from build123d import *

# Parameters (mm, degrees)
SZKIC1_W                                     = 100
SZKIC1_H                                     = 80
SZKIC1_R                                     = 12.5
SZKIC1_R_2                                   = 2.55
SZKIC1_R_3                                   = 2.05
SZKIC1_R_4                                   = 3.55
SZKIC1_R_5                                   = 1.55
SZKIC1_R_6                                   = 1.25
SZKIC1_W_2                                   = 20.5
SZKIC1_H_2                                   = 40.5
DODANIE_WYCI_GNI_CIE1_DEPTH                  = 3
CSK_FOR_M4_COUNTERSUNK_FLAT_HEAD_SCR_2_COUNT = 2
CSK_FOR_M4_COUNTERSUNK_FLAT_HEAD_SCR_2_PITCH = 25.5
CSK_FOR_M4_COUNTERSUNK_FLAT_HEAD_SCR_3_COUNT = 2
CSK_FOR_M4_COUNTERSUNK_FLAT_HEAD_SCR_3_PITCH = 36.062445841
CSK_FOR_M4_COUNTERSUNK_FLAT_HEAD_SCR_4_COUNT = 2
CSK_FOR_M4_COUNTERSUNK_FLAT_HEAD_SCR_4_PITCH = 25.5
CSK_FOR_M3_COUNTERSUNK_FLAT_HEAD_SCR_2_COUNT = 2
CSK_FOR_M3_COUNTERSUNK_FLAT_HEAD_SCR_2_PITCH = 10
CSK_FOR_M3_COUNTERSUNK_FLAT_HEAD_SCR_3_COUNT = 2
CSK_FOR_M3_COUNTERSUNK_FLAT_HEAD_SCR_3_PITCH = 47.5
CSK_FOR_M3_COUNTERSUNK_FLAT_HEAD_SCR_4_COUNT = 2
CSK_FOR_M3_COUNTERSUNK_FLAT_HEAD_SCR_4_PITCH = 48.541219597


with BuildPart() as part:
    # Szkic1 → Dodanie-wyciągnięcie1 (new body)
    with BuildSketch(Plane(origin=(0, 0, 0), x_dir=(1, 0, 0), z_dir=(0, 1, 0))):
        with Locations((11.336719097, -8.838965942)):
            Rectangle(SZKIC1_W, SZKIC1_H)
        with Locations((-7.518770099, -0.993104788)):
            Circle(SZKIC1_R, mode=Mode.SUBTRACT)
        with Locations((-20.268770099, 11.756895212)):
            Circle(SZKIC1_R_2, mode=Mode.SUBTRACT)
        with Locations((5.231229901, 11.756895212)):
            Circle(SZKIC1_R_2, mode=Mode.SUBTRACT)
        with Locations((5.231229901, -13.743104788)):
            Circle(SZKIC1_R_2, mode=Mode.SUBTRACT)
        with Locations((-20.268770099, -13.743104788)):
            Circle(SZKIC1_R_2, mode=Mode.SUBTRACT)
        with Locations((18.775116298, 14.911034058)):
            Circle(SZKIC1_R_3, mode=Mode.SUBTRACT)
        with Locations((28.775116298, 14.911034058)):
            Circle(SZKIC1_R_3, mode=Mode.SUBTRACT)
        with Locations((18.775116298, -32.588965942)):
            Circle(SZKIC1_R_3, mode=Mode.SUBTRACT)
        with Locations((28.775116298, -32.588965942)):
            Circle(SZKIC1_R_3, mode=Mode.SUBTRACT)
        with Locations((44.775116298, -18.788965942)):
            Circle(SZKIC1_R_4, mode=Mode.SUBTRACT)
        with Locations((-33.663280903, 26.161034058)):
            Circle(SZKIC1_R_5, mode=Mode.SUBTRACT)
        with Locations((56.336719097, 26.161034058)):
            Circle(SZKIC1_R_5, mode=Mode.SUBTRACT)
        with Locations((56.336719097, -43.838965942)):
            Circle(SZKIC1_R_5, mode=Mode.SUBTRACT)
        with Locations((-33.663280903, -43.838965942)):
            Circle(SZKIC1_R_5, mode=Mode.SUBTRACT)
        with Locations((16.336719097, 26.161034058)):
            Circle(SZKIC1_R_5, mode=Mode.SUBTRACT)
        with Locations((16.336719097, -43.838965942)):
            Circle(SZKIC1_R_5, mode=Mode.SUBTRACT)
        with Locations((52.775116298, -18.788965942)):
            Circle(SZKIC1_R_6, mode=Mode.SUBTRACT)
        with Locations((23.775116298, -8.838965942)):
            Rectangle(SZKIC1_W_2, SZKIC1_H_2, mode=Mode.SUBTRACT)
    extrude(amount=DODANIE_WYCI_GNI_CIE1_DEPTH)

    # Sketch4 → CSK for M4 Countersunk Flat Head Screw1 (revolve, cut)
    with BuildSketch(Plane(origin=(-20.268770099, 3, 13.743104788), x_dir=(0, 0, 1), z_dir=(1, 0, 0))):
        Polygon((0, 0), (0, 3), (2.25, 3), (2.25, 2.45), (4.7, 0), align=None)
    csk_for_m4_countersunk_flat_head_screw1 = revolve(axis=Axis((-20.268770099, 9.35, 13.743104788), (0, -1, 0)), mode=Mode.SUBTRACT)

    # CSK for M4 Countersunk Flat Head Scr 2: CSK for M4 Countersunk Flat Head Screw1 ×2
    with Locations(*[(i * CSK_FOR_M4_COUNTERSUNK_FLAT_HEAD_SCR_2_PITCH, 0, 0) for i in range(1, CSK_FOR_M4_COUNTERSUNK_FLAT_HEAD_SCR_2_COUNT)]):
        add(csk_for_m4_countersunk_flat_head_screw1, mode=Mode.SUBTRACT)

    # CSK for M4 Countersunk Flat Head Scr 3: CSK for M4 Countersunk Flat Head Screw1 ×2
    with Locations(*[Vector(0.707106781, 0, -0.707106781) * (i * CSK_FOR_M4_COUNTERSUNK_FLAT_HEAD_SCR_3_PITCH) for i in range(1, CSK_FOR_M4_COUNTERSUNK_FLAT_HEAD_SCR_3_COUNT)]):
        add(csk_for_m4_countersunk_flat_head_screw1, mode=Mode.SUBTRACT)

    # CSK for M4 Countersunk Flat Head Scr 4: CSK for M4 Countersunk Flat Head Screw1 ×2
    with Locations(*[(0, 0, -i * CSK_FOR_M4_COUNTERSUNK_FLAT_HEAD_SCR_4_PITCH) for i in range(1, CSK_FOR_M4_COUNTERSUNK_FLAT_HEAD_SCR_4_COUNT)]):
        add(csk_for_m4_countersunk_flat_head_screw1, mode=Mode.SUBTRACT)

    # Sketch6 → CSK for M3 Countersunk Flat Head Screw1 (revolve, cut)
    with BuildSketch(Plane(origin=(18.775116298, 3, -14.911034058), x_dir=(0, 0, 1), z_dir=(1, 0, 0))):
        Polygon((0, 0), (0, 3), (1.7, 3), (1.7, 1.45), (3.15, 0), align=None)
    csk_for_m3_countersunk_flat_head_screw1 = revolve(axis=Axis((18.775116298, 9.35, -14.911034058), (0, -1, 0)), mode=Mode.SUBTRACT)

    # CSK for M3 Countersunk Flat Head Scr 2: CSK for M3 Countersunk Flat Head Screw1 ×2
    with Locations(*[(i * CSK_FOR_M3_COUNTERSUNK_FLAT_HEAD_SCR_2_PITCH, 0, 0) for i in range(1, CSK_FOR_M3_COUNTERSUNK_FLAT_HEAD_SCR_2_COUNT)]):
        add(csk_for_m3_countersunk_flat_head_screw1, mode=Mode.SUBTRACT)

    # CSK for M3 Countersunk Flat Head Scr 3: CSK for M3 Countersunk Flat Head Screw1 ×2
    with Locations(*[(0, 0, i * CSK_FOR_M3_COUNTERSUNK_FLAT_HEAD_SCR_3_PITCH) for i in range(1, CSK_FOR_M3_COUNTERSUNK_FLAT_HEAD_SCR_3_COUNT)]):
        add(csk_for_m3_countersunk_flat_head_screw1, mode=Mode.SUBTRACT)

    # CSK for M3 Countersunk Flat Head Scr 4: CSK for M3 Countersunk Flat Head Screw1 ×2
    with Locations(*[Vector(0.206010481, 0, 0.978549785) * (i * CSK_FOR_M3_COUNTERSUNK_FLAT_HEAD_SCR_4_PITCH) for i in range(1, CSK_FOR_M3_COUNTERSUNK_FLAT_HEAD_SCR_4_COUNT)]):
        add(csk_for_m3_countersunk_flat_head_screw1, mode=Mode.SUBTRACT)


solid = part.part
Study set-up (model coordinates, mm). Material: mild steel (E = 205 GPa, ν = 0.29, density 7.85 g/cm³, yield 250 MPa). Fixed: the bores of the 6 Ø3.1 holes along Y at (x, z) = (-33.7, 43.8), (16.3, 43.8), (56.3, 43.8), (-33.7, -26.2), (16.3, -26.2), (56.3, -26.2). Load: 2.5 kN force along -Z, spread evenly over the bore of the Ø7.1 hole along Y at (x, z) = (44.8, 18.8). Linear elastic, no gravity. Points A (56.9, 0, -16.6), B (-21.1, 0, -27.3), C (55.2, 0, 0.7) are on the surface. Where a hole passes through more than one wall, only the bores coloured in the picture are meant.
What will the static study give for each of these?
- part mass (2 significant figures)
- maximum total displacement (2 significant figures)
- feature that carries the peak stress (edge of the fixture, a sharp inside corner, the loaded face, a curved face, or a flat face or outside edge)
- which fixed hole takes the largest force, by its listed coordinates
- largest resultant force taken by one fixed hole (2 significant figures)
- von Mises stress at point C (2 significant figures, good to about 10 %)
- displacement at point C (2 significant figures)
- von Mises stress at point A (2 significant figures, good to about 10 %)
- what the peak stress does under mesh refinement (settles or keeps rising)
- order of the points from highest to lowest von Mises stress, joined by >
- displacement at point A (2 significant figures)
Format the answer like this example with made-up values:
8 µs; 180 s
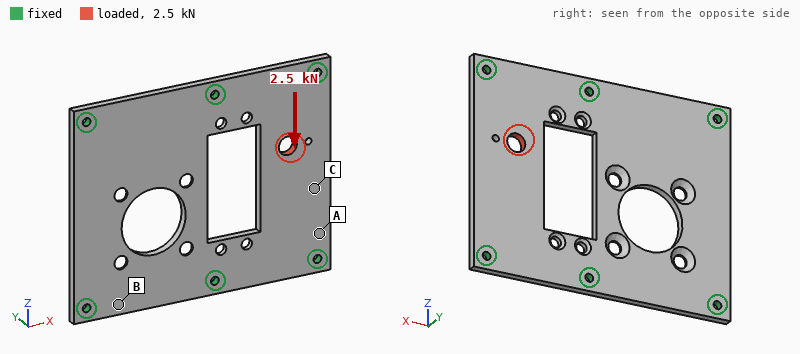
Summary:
150 g; 4.7 µm; edge of the fixture; (56.3, 43.8); 1.2 kN; 12 MPa; 2.3 µm; 19 MPa; keeps rising; A > C > B; 1.1 µm
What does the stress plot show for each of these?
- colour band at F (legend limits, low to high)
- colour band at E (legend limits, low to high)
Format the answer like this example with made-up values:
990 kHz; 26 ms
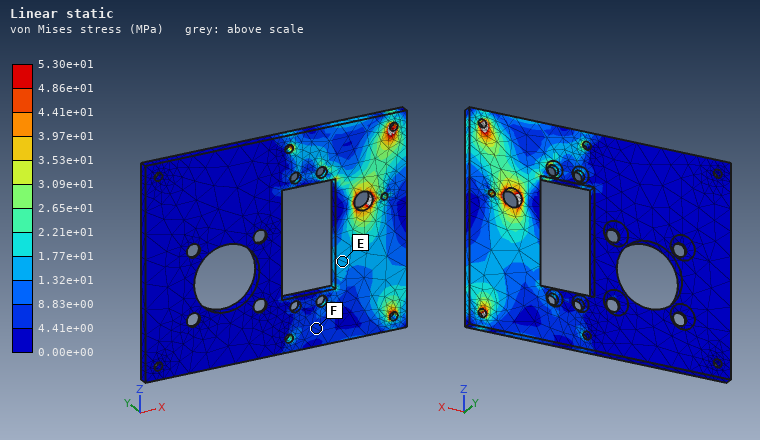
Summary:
4.41e+00 to 8.83e+00 MPa; 1.32e+01 to 1.77e+01 MPa
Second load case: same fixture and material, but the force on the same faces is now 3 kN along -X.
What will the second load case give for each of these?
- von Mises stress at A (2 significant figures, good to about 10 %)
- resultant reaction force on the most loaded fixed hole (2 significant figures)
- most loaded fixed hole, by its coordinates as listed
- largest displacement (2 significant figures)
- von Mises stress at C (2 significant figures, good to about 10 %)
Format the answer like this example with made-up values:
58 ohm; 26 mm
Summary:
19 MPa; 1.3 kN; (56.3, 43.8); 13 µm; 23 MPa
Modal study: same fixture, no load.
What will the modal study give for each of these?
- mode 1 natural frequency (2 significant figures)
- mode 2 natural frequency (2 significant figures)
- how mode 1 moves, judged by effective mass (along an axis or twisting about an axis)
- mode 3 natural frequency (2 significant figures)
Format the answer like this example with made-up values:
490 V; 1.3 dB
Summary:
2700 Hz; 3000 Hz; along Y; 4300 Hz
